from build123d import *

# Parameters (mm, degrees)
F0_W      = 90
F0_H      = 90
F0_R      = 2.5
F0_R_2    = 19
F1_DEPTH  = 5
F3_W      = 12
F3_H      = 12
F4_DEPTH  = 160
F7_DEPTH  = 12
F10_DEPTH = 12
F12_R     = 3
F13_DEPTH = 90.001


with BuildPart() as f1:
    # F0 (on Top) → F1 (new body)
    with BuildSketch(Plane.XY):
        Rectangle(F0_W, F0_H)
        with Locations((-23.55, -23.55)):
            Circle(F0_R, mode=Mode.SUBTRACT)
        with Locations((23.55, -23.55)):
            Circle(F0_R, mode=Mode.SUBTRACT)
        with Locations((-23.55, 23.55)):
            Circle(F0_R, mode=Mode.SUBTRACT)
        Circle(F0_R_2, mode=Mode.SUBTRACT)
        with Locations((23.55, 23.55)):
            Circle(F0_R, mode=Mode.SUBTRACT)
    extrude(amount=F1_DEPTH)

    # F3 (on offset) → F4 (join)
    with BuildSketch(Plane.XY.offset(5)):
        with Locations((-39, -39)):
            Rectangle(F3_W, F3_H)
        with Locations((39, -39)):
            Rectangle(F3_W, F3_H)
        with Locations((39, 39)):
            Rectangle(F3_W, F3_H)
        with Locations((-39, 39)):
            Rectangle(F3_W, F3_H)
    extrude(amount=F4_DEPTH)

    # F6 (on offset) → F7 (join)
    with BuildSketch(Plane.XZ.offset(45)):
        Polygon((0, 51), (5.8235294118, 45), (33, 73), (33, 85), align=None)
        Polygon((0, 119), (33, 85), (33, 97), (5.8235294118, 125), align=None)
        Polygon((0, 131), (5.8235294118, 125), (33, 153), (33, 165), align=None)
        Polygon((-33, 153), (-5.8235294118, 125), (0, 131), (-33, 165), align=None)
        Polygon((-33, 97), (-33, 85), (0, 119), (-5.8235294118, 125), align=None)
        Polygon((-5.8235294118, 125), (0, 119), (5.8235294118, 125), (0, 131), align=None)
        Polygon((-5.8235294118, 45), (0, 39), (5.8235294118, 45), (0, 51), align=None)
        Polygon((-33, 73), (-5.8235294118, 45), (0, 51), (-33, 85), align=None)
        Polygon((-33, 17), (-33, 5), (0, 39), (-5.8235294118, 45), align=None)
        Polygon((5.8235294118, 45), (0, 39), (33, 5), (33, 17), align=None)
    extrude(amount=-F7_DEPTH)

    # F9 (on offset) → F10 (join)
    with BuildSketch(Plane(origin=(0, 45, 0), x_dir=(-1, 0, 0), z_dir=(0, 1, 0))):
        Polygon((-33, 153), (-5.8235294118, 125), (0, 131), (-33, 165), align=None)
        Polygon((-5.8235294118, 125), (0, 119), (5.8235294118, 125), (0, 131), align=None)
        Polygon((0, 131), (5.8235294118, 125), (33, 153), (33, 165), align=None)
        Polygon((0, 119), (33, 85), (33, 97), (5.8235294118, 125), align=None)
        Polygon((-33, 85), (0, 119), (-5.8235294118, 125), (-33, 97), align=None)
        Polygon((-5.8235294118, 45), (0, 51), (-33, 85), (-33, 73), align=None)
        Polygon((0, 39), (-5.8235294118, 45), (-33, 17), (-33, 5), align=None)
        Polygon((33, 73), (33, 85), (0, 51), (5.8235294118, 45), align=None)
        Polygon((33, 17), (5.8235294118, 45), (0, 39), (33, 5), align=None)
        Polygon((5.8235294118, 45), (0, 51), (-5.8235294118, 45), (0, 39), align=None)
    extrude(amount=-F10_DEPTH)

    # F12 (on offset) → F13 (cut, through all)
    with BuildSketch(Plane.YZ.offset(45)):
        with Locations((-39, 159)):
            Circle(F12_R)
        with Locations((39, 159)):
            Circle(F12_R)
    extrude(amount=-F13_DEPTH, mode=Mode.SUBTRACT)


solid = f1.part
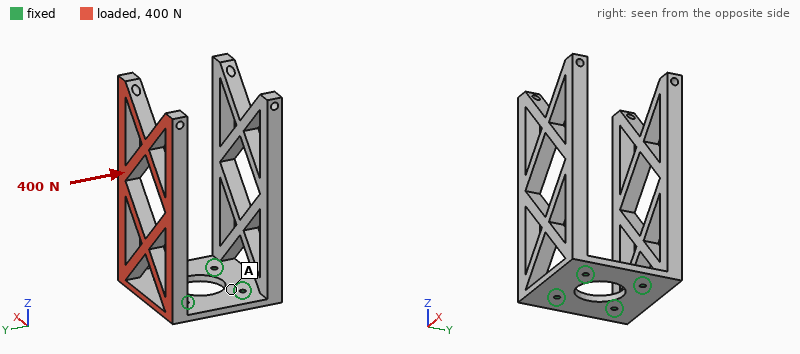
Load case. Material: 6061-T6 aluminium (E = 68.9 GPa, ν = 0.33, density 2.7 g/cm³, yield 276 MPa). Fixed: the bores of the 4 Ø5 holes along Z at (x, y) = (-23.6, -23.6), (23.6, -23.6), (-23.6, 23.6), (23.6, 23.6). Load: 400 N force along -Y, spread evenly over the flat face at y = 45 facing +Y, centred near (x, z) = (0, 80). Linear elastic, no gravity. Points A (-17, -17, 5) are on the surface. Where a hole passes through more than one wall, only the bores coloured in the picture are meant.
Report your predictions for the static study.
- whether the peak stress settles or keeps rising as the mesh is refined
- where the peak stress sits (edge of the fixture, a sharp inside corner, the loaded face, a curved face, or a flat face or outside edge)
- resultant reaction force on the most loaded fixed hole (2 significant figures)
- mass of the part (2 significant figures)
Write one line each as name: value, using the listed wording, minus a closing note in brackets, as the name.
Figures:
whether the peak stress settles or keeps rising as the mesh is refined: keeps rising
where the peak stress sits: edge of the fixture
resultant reaction force on the most loaded fixed hole: 190 N
mass of the part: 530 g
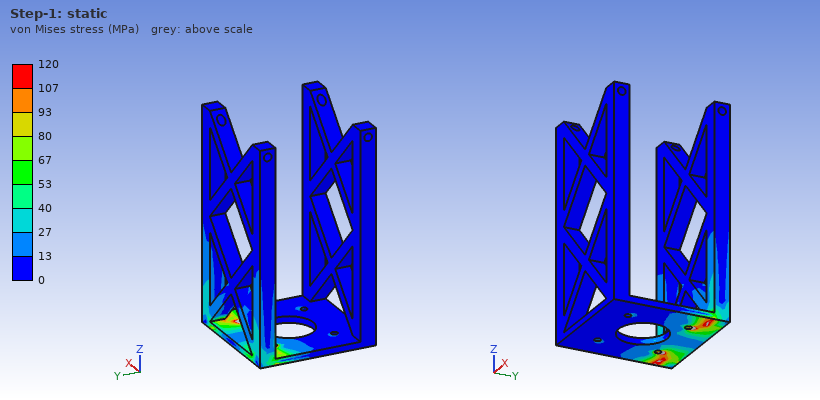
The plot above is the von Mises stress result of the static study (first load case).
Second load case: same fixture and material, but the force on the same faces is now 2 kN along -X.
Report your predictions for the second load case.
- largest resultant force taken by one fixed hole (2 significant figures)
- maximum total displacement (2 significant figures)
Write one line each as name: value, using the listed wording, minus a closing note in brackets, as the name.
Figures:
largest resultant force taken by one fixed hole: 2.9 kN
maximum total displacement: 0.71 mm
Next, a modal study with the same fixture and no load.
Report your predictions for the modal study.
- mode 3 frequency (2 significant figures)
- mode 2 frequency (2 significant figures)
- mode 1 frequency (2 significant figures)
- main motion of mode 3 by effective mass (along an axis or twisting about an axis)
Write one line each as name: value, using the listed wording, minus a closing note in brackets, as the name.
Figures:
mode 3 frequency: 620 Hz
mode 2 frequency: 170 Hz
mode 1 frequency: 170 Hz
main motion of mode 3 by effective mass: along X
